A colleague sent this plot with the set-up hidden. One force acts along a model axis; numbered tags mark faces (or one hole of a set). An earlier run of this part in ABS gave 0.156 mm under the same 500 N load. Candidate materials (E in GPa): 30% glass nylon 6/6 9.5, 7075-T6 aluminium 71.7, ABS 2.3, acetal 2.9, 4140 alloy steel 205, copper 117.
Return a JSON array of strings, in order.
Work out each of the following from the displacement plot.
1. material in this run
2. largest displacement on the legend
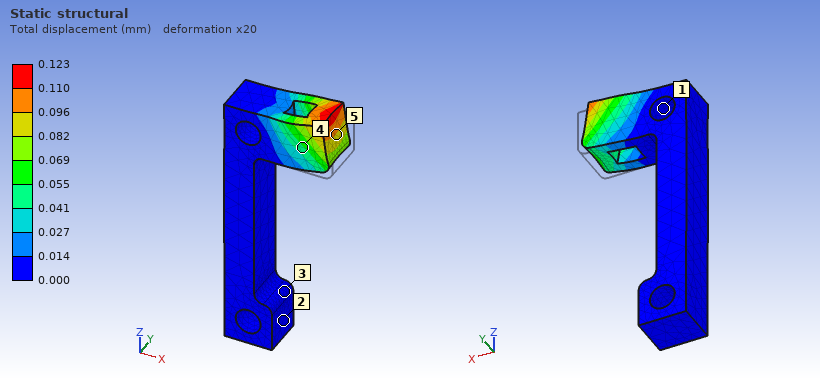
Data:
["acetal", "0.123 mm"]
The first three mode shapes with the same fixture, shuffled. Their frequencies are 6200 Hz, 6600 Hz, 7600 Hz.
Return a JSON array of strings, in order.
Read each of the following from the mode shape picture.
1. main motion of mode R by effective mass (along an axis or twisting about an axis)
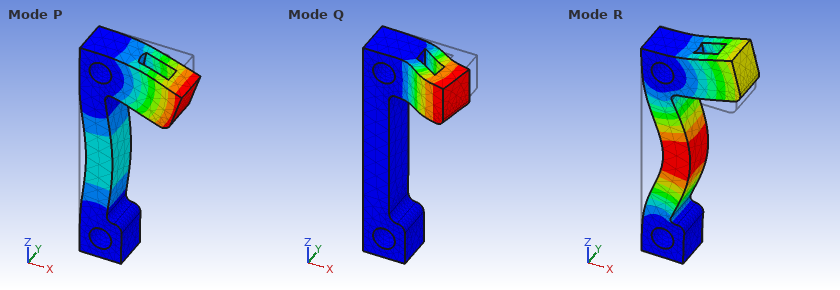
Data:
["along X"]
